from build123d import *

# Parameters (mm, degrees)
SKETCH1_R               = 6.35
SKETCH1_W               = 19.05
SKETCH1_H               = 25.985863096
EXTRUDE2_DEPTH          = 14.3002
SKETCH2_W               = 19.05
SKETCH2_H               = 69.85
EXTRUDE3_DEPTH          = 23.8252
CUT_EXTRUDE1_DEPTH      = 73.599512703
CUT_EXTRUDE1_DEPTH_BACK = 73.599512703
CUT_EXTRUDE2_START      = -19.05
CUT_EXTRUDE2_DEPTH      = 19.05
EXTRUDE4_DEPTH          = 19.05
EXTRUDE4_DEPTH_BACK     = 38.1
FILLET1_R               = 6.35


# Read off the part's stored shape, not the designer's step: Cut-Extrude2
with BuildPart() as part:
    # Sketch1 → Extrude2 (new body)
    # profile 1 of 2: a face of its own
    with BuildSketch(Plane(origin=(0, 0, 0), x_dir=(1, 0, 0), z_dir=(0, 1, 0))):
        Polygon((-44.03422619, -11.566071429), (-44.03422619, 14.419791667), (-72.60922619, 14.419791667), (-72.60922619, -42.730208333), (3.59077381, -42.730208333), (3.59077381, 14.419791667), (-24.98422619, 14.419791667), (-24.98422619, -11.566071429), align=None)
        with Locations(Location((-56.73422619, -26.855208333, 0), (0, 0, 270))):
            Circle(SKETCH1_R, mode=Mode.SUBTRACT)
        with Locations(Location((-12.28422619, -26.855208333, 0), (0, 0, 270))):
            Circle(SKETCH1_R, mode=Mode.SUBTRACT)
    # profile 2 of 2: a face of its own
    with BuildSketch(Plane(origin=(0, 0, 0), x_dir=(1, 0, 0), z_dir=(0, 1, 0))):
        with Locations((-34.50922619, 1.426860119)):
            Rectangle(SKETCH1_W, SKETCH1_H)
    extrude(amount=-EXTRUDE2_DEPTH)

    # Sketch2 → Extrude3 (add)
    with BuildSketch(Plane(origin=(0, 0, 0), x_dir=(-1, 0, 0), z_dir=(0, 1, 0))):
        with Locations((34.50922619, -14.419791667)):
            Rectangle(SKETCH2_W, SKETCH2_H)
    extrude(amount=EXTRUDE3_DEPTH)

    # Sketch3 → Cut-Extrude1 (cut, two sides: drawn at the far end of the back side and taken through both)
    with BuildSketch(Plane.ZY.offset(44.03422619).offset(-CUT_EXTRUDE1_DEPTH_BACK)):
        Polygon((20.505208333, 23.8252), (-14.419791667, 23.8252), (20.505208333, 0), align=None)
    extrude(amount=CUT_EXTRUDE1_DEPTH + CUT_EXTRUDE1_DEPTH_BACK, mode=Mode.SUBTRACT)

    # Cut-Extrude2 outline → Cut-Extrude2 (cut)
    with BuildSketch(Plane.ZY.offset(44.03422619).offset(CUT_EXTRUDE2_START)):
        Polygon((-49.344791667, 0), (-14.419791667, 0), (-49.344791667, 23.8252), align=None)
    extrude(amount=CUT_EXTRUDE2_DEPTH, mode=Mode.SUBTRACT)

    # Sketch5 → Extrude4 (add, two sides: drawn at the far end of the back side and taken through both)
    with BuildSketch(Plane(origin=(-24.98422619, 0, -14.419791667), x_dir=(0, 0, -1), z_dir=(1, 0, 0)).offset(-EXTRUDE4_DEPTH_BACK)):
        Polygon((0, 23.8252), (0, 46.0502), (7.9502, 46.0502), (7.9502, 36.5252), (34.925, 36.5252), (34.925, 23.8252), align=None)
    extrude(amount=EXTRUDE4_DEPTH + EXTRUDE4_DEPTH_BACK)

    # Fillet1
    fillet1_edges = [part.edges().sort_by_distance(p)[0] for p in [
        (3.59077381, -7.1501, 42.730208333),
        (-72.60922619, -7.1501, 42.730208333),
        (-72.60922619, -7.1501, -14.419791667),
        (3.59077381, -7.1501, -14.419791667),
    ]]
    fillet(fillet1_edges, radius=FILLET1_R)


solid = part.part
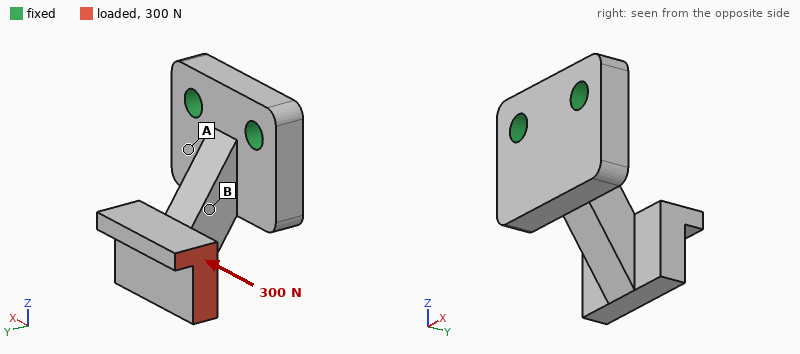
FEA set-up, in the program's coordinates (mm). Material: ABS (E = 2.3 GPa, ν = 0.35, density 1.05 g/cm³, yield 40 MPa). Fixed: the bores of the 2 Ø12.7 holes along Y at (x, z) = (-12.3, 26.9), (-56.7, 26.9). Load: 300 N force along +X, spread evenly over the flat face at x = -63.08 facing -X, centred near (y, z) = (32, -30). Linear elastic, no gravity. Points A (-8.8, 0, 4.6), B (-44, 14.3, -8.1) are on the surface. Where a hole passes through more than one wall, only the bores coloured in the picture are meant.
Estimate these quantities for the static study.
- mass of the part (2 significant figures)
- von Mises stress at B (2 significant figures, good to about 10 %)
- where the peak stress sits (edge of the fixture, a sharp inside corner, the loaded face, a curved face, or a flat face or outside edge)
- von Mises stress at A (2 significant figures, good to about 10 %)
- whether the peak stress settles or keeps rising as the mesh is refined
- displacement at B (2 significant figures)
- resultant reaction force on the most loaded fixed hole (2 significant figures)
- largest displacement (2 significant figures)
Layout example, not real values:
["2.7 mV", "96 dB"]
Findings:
["110 g", "6.4 MPa", "a sharp inside corner", "1.3 MPa", "keeps rising", "0.17 mm", "450 N", "0.76 mm"]
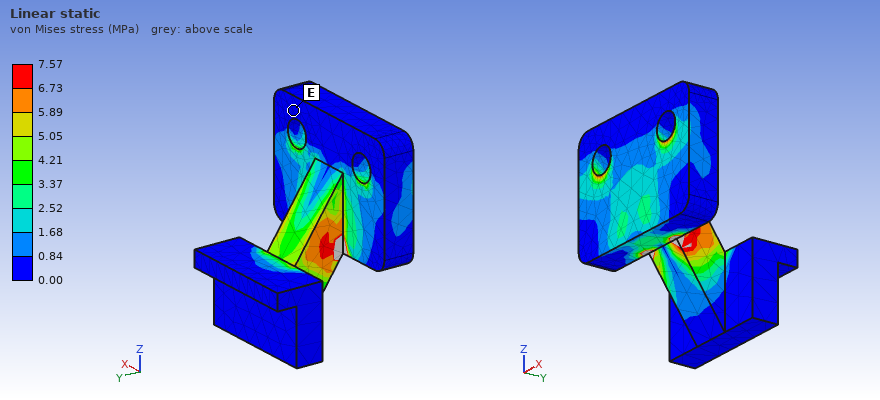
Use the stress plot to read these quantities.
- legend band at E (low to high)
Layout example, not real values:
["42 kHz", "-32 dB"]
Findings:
["0.00 to 0.84 MPa"]
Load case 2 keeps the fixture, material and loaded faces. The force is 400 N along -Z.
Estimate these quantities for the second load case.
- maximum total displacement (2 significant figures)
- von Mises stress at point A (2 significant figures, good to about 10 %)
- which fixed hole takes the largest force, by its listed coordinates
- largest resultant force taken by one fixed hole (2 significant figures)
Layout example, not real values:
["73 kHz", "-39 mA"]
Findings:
["1.6 mm", "2.4 MPa", "(-56.7, 26.9)", "440 N"]
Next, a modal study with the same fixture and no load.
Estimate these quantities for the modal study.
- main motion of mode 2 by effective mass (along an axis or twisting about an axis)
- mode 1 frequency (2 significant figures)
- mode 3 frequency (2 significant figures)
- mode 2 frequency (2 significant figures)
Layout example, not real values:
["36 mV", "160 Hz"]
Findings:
["along X", "490 Hz", "1000 Hz", "620 Hz"]
